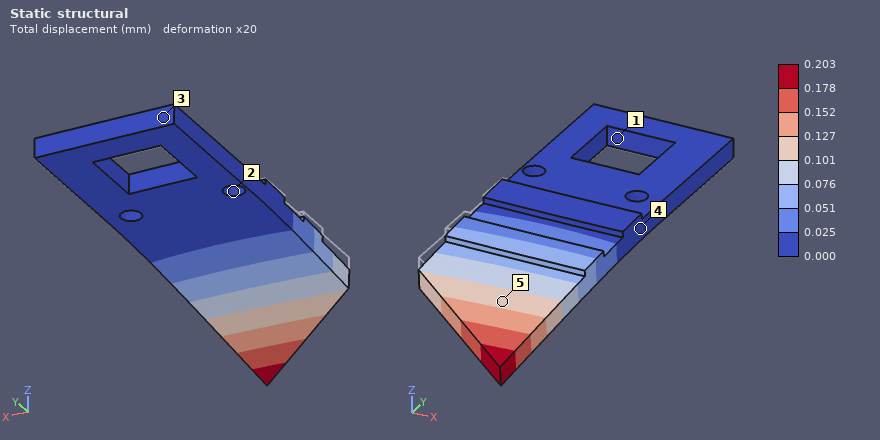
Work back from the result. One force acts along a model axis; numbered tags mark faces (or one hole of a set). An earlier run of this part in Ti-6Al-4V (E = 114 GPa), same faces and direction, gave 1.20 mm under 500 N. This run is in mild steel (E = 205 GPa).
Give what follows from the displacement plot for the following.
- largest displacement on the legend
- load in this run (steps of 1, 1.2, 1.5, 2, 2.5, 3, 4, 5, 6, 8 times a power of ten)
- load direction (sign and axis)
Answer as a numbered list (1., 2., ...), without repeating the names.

1. 0.203 mm
2. 150 N
3. -Z
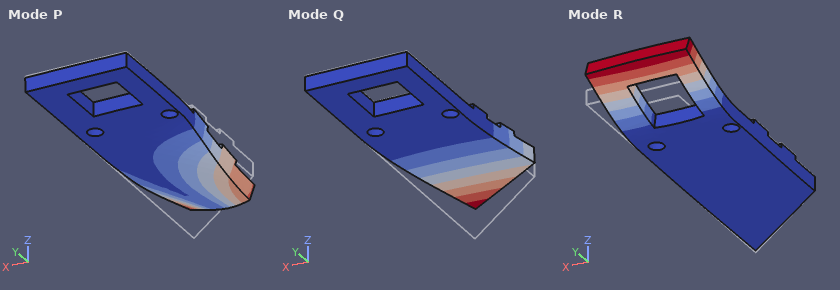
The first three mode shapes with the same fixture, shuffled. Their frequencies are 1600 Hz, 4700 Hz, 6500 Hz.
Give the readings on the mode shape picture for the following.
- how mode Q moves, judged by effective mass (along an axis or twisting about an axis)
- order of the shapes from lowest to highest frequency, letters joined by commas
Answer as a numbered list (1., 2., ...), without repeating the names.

1. along Z
2. Q, R, P
